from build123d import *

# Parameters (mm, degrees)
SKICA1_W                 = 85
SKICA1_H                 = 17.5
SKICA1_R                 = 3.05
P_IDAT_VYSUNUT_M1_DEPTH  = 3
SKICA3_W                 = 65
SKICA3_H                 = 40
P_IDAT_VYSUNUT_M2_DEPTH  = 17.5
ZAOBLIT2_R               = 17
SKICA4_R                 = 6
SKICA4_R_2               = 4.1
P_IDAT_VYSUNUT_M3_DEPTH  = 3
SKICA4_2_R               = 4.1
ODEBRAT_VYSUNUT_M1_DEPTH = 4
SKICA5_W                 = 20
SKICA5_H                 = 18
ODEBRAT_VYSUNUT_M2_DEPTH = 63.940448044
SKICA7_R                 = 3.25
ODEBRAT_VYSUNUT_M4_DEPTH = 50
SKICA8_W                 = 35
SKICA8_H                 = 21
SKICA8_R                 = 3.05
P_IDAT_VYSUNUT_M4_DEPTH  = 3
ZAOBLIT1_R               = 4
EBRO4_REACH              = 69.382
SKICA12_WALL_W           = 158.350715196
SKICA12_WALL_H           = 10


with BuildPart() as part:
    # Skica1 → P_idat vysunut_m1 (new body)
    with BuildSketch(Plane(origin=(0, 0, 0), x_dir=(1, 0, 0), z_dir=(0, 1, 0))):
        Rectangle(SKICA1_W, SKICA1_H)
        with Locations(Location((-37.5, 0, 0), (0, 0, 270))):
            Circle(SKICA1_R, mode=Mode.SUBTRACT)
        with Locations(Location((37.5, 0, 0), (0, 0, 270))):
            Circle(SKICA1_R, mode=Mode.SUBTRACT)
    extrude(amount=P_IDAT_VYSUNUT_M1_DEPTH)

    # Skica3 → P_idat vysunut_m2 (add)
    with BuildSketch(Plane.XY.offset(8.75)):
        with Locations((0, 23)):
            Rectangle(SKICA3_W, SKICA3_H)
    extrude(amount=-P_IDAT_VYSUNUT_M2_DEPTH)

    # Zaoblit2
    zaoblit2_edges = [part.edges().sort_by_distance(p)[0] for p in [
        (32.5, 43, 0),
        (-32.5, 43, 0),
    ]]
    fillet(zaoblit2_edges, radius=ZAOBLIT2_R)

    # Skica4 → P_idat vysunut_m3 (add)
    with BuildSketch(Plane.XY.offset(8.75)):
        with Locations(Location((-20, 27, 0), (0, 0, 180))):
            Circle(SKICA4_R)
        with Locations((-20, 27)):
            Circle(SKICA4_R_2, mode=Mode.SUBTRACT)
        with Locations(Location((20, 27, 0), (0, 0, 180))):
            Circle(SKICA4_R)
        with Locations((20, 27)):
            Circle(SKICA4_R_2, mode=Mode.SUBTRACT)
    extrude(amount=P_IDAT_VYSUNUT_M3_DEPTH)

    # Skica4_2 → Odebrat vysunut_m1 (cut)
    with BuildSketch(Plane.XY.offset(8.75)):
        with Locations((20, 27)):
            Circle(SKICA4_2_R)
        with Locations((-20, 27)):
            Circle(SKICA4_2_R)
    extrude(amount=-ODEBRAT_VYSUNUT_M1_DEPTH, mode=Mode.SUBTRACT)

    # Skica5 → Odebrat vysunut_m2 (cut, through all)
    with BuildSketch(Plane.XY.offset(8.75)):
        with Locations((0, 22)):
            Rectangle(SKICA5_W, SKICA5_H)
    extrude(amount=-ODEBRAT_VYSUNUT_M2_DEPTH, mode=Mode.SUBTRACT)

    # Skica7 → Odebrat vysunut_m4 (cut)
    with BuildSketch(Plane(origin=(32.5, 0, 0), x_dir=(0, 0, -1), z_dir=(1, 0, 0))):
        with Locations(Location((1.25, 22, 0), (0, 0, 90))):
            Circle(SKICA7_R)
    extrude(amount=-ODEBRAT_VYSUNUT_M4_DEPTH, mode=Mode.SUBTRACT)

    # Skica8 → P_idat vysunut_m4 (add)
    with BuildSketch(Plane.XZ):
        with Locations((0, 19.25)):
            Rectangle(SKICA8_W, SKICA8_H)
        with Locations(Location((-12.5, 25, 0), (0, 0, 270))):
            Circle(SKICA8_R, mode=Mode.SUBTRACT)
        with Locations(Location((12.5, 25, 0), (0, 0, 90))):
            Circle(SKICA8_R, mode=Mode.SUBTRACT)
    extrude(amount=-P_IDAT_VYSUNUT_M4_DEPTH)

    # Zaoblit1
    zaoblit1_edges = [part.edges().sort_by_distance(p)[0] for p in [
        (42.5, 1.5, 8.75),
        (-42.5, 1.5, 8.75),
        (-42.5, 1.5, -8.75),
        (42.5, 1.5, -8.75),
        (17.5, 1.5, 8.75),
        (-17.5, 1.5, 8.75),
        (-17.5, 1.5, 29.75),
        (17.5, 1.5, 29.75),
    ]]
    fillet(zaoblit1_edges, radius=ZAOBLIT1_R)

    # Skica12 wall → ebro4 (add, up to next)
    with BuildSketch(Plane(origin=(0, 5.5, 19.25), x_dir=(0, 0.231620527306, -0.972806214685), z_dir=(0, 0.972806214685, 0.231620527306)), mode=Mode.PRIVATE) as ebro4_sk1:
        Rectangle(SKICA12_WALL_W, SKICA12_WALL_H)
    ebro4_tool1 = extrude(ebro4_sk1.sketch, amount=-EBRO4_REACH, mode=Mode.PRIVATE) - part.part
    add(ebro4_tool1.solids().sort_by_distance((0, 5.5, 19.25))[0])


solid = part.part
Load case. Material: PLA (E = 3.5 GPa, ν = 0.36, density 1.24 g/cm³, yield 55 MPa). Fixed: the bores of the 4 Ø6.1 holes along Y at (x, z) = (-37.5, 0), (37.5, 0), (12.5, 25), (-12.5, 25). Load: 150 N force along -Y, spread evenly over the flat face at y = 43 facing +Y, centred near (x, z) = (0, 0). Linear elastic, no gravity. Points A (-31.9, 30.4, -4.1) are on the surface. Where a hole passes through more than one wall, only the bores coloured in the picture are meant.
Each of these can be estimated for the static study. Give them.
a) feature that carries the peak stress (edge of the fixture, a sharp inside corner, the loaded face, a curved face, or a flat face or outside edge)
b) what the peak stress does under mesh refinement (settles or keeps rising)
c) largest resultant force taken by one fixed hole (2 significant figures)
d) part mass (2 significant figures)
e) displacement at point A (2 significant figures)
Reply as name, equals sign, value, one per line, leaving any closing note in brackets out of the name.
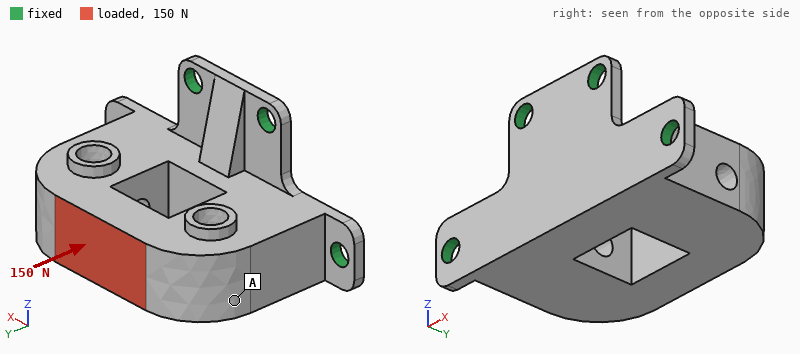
feature that carries the peak stress = edge of the fixture
what the peak stress does under mesh refinement = keeps rising
largest resultant force taken by one fixed hole = 83 N
part mass = 53 g
displacement at point A = 23 µm
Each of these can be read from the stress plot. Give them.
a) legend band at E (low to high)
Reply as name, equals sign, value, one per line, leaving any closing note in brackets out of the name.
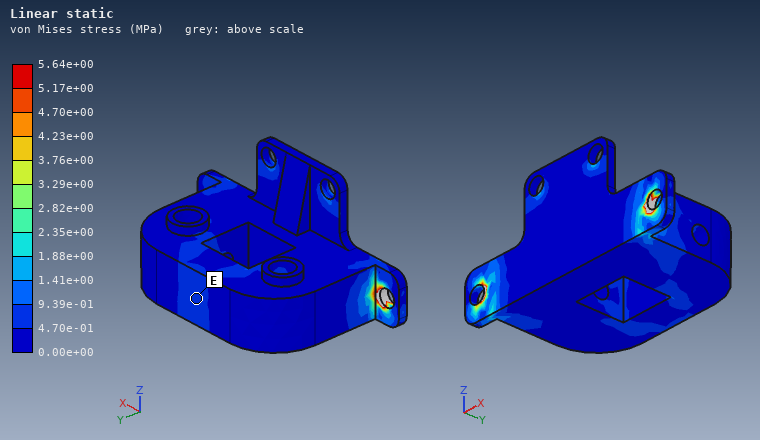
legend band at E = 4.70e-01 to 9.39e-01 MPa
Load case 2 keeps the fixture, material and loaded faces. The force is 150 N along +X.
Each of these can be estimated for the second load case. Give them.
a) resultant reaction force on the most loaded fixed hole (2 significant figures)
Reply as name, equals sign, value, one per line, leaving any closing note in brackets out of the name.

resultant reaction force on the most loaded fixed hole = 110 N
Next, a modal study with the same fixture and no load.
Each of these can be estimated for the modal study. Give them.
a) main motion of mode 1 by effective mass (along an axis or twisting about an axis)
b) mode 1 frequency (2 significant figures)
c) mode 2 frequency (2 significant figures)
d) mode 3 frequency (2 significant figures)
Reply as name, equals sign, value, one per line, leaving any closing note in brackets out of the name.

main motion of mode 1 by effective mass = along Z
mode 1 frequency = 720 Hz
mode 2 frequency = 2400 Hz
mode 3 frequency = 2400 Hz
